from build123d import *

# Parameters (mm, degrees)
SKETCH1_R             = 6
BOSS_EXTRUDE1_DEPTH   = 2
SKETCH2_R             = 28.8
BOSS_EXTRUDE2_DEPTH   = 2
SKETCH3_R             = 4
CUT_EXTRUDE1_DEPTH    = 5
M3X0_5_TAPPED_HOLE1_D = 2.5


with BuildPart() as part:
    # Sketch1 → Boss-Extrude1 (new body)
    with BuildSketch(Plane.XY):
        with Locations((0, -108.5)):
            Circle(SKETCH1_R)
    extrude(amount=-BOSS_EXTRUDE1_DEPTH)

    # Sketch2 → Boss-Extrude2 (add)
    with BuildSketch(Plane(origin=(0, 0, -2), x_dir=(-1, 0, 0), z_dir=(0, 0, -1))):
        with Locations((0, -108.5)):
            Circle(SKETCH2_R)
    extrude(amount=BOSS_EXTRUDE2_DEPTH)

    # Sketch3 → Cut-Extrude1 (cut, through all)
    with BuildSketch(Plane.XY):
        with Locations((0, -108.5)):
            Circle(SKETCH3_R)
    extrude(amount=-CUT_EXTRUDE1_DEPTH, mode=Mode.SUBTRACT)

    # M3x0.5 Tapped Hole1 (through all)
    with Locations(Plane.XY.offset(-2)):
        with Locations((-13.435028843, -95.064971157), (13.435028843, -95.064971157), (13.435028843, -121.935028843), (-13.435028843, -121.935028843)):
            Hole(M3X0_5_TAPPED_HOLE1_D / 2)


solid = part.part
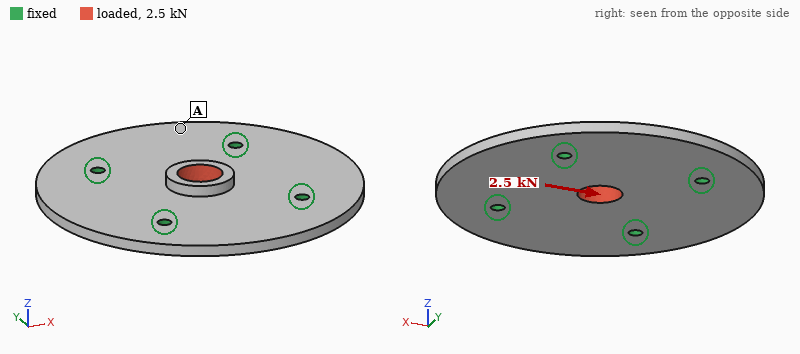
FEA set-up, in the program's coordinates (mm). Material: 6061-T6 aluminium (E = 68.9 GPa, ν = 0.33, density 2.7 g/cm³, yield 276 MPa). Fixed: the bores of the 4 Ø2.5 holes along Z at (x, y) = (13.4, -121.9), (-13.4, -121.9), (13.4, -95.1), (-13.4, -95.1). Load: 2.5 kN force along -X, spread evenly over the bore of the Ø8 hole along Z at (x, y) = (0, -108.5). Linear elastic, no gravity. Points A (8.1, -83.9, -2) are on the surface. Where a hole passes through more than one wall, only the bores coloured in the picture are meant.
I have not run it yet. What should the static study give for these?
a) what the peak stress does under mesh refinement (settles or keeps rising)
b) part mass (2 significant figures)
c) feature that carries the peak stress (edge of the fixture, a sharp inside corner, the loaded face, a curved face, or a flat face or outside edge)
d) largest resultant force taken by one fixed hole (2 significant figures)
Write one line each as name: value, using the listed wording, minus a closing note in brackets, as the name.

what the peak stress does under mesh refinement: keeps rising
part mass: 14 g
feature that carries the peak stress: edge of the fixture
largest resultant force taken by one fixed hole: 650 N
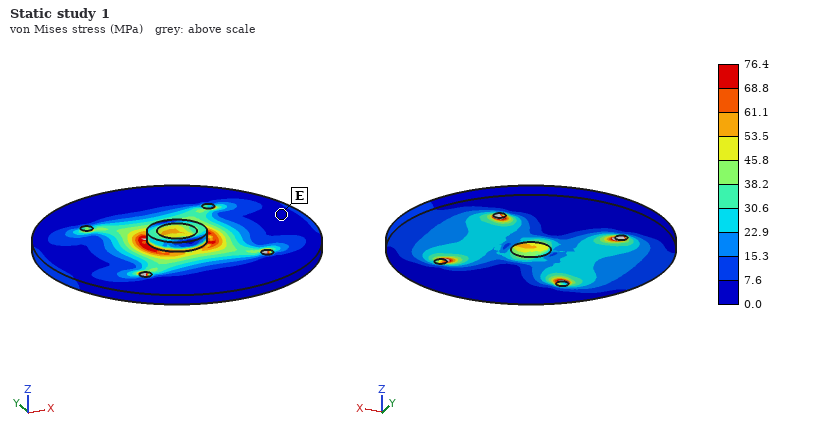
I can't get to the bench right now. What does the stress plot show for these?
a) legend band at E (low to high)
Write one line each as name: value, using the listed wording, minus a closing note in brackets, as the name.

legend band at E: 0.0 to 7.6 MPa
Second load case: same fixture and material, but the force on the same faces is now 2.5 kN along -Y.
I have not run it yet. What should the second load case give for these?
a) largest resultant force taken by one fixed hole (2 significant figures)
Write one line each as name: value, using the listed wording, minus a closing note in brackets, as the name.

largest resultant force taken by one fixed hole: 650 N
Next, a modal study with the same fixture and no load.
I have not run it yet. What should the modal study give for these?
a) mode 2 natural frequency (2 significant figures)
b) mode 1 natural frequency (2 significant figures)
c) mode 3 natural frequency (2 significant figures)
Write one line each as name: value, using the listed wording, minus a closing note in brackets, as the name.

mode 2 natural frequency: 7100 Hz
mode 1 natural frequency: 6400 Hz
mode 3 natural frequency: 7100 Hz
